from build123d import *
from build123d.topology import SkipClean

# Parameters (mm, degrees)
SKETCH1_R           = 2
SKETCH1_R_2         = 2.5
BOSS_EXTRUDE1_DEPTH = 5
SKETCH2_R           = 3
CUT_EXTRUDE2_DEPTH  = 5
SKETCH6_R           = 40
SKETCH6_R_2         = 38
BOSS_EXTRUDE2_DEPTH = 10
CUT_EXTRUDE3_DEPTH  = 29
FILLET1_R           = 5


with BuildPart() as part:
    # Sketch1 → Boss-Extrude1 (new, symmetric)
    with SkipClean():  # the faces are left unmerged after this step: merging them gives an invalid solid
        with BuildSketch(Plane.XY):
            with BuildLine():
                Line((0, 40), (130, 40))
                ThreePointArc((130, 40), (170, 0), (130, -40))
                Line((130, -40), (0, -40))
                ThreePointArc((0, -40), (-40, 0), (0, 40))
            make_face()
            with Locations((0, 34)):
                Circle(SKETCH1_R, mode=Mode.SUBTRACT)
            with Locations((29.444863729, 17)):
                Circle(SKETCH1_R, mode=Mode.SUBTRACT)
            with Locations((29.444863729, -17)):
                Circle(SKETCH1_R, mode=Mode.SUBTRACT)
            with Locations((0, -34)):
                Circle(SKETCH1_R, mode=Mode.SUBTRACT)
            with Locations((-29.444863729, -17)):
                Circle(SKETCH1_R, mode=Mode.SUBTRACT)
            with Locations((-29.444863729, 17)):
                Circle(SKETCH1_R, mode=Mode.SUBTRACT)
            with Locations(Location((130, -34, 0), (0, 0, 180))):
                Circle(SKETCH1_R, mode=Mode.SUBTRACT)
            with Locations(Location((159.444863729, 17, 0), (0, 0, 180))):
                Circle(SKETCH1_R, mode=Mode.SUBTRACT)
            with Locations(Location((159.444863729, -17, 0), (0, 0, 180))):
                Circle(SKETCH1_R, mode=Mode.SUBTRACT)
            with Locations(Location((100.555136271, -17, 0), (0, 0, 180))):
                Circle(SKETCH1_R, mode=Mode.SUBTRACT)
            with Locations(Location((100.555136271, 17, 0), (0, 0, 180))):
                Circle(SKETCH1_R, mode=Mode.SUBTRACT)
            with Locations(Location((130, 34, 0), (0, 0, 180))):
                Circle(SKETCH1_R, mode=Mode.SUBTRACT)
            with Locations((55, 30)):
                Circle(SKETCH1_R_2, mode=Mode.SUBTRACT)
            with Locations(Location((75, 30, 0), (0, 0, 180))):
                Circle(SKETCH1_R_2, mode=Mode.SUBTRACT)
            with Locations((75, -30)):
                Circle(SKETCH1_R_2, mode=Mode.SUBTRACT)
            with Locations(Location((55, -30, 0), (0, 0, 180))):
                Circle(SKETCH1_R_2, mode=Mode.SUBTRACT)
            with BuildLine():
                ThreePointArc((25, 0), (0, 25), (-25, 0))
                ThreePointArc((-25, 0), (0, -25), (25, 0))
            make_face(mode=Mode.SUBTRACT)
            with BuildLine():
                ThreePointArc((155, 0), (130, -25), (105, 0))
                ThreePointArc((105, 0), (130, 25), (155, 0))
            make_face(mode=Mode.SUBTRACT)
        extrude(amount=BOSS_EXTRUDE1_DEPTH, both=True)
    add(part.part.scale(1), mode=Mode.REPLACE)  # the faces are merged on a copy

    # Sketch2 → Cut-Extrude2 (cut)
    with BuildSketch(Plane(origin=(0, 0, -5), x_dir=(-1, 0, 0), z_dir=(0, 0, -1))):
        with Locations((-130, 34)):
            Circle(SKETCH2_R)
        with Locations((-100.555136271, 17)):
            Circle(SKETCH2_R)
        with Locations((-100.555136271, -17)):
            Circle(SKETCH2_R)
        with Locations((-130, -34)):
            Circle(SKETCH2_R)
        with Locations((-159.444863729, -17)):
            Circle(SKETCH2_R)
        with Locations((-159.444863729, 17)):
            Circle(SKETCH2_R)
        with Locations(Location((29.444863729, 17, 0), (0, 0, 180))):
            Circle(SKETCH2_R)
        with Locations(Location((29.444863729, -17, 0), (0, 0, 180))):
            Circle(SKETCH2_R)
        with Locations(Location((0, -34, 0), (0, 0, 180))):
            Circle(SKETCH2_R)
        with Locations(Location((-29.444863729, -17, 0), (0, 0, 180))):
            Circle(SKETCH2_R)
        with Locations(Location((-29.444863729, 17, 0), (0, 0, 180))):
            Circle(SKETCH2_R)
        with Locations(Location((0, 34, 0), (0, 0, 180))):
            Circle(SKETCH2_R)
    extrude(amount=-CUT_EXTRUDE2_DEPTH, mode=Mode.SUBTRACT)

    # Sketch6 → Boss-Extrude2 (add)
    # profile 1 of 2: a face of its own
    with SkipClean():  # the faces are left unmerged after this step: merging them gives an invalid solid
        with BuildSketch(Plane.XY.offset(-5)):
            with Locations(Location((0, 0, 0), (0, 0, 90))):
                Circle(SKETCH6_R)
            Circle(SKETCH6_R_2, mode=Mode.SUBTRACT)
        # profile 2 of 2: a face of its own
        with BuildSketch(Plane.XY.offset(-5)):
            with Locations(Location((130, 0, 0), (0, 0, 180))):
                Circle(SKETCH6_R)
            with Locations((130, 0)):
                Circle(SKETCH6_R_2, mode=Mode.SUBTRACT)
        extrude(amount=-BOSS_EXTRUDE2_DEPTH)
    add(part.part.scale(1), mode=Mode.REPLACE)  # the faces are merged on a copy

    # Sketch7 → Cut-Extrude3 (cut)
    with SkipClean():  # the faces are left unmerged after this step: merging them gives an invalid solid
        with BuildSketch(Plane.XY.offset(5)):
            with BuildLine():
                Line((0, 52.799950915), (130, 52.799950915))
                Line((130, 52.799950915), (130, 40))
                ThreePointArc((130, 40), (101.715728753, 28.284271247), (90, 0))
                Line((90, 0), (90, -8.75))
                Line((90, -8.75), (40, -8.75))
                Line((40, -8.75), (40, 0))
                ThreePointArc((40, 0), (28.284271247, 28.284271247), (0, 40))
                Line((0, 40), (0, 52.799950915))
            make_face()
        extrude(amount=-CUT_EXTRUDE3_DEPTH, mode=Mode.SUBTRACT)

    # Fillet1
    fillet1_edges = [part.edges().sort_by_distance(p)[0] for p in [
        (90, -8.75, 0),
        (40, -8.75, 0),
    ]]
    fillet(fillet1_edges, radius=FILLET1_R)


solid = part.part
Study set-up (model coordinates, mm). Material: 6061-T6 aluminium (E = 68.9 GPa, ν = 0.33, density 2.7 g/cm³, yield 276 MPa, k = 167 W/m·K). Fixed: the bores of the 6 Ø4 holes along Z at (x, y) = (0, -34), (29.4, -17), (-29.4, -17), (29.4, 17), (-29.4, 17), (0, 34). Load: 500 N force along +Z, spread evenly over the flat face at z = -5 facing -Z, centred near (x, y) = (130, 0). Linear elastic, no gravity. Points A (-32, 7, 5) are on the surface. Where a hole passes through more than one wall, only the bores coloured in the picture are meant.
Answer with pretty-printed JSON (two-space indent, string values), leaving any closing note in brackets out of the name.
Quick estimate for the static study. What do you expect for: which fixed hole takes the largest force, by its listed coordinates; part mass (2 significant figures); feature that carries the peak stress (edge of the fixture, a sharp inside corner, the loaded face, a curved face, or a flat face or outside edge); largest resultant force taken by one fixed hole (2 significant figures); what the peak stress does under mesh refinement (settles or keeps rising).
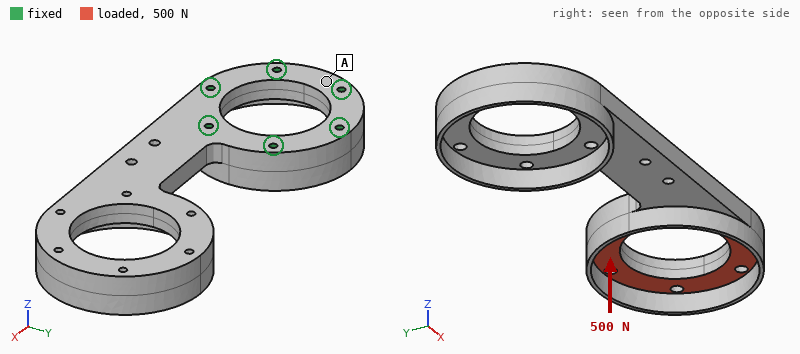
{
  "which fixed hole takes the largest force, by its listed coordinates": "(29.4, -17)",
  "part mass": "250 g",
  "feature that carries the peak stress": "edge of the fixture",
  "largest resultant force taken by one fixed hole": "2.1 kN",
  "what the peak stress does under mesh refinement": "keeps rising"
}
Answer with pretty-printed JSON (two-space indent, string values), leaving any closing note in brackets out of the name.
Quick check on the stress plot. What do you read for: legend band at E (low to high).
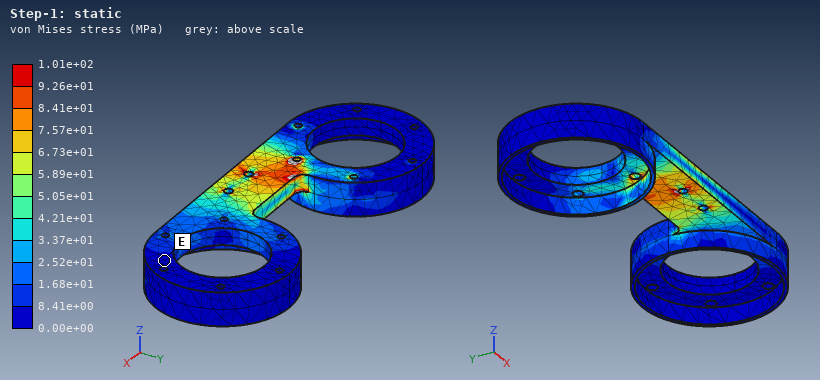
{
  "legend band at E": "0.00e+00 to 8.41e+00 MPa"
}
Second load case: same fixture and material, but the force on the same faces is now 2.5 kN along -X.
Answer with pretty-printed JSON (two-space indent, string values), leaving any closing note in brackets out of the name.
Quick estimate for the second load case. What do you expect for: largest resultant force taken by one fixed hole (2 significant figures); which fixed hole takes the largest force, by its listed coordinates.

{
  "largest resultant force taken by one fixed hole": "2.1 kN",
  "which fixed hole takes the largest force, by its listed coordinates": "(29.4, -17)"
}
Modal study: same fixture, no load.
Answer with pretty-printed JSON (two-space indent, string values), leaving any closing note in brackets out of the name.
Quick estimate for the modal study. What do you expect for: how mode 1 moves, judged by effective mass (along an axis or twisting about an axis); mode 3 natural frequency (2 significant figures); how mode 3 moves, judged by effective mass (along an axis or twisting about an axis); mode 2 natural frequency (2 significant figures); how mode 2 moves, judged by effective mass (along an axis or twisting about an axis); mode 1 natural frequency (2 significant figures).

{
  "how mode 1 moves, judged by effective mass": "along Z",
  "mode 3 natural frequency": "960 Hz",
  "how mode 3 moves, judged by effective mass": "twisting about X",
  "mode 2 natural frequency": "850 Hz",
  "how mode 2 moves, judged by effective mass": "along Y",
  "mode 1 natural frequency": "310 Hz"
}
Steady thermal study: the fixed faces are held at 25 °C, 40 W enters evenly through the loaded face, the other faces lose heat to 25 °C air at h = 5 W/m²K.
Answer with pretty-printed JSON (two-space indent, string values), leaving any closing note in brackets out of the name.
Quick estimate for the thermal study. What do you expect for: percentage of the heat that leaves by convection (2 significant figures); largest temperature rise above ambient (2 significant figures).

{
  "percentage of the heat that leaves by convection": "14 %",
  "largest temperature rise above ambient": "80 K"
}
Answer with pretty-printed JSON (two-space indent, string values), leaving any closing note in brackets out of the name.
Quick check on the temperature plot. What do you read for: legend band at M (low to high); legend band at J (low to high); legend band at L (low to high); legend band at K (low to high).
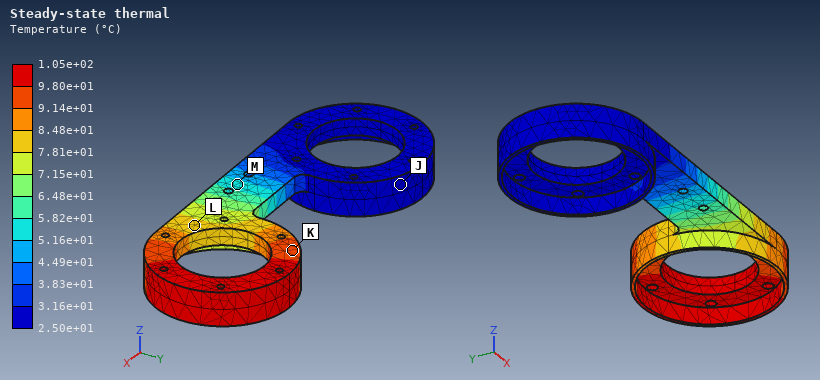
{
  "legend band at M": "5.16e+01 to 5.82e+01 °C",
  "legend band at J": "2.50e+01 to 3.16e+01 °C",
  "legend band at L": "7.81e+01 to 8.48e+01 °C",
  "legend band at K": "9.14e+01 to 9.80e+01 °C"
}
